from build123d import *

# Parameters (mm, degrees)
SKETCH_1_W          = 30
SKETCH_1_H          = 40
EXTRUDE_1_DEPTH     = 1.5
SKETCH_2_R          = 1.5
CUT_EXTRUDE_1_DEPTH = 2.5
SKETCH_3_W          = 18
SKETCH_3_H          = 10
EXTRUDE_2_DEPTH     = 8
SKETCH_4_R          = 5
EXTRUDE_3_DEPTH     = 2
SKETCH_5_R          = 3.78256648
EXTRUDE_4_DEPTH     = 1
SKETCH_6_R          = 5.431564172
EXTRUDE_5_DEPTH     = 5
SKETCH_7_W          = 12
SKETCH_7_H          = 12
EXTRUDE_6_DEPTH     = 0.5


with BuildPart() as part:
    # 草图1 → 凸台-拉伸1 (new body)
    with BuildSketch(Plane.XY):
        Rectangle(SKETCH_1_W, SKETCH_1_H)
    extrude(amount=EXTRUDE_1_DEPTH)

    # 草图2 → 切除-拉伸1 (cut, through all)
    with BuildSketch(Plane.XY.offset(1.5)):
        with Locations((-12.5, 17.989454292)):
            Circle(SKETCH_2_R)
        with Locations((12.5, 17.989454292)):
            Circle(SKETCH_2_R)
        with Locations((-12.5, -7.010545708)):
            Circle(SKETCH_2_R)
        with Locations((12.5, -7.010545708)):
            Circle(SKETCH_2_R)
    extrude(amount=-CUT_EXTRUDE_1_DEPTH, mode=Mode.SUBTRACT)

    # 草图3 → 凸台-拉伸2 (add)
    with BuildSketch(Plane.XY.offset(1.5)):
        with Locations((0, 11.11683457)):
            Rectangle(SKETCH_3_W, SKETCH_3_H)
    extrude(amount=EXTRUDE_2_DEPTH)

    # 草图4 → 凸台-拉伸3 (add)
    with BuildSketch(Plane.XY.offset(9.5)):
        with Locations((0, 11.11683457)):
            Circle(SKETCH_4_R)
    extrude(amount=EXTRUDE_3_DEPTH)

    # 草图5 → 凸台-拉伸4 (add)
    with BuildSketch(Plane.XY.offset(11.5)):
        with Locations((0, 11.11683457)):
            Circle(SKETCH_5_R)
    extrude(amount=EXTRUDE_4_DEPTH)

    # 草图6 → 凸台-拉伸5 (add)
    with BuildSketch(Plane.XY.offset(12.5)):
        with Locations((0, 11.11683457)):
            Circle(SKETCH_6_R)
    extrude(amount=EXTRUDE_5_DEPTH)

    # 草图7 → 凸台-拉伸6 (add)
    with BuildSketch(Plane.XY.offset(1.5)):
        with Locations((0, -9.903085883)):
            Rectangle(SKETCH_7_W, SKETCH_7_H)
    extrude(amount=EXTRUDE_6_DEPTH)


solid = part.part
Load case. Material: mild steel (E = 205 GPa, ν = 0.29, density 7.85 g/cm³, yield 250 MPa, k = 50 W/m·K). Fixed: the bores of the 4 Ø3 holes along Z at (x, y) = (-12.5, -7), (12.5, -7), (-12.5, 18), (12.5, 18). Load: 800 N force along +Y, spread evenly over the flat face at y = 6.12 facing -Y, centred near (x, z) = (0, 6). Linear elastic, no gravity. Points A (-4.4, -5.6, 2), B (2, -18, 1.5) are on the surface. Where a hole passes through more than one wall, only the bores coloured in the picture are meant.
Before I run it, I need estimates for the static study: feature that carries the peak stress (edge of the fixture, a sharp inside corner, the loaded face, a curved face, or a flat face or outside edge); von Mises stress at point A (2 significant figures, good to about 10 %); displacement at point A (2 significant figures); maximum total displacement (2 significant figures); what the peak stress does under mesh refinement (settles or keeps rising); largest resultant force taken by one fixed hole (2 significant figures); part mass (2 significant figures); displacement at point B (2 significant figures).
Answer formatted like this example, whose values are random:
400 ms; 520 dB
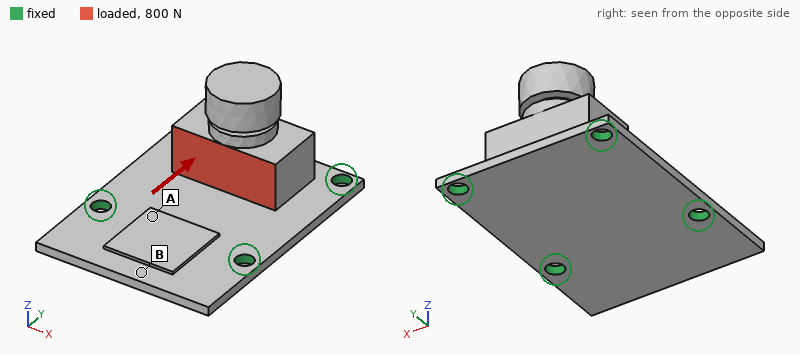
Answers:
edge of the fixture; 28 MPa; 5.7 µm; 38 µm; keeps rising; 260 N; 31 g; 6.5 µm
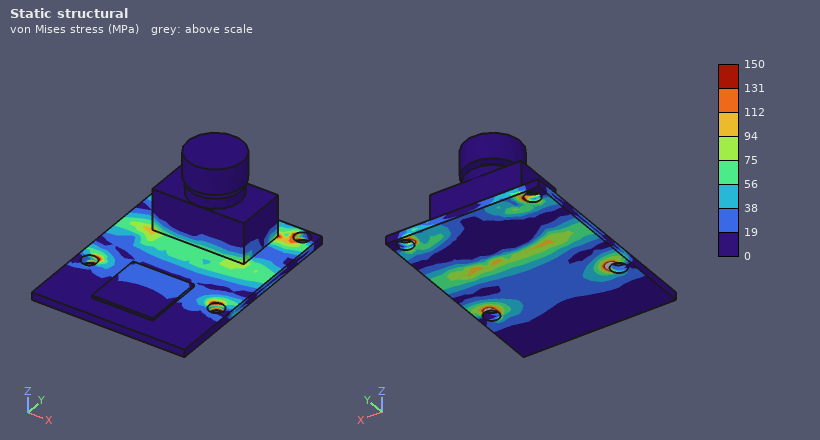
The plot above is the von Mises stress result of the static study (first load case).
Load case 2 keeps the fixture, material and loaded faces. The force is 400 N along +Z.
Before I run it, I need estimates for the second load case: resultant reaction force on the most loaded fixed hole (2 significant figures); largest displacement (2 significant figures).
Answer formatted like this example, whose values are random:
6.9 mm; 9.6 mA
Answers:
110 N; 37 µm
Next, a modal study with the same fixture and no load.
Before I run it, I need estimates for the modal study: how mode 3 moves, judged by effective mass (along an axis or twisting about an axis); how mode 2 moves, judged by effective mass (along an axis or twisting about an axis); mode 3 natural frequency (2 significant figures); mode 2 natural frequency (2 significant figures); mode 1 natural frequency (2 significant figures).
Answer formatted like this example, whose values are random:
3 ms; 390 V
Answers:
along X; along Z; 11 kHz; 6900 Hz; 4900 Hz
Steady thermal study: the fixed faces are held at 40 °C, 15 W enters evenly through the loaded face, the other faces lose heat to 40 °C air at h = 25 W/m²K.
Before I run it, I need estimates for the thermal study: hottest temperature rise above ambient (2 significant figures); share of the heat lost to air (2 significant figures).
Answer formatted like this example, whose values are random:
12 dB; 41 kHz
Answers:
51 K; 13 %
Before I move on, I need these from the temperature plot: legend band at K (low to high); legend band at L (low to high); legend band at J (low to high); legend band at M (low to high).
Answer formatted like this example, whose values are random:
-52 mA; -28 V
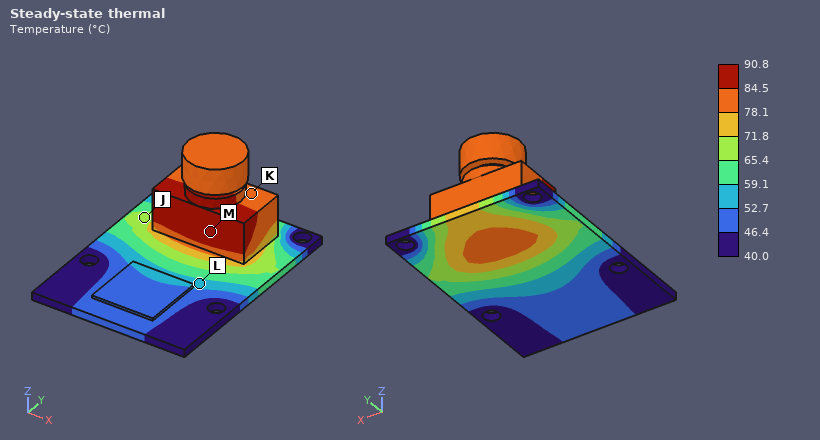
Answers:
78.1 to 84.5 °C; 52.7 to 59.1 °C; 65.4 to 71.8 °C; 84.5 to 90.8 °C
